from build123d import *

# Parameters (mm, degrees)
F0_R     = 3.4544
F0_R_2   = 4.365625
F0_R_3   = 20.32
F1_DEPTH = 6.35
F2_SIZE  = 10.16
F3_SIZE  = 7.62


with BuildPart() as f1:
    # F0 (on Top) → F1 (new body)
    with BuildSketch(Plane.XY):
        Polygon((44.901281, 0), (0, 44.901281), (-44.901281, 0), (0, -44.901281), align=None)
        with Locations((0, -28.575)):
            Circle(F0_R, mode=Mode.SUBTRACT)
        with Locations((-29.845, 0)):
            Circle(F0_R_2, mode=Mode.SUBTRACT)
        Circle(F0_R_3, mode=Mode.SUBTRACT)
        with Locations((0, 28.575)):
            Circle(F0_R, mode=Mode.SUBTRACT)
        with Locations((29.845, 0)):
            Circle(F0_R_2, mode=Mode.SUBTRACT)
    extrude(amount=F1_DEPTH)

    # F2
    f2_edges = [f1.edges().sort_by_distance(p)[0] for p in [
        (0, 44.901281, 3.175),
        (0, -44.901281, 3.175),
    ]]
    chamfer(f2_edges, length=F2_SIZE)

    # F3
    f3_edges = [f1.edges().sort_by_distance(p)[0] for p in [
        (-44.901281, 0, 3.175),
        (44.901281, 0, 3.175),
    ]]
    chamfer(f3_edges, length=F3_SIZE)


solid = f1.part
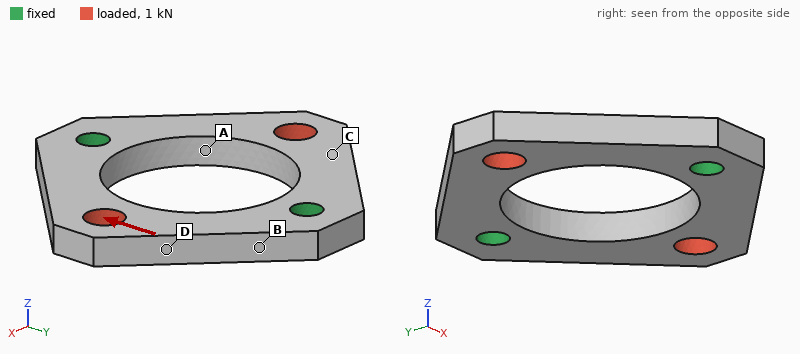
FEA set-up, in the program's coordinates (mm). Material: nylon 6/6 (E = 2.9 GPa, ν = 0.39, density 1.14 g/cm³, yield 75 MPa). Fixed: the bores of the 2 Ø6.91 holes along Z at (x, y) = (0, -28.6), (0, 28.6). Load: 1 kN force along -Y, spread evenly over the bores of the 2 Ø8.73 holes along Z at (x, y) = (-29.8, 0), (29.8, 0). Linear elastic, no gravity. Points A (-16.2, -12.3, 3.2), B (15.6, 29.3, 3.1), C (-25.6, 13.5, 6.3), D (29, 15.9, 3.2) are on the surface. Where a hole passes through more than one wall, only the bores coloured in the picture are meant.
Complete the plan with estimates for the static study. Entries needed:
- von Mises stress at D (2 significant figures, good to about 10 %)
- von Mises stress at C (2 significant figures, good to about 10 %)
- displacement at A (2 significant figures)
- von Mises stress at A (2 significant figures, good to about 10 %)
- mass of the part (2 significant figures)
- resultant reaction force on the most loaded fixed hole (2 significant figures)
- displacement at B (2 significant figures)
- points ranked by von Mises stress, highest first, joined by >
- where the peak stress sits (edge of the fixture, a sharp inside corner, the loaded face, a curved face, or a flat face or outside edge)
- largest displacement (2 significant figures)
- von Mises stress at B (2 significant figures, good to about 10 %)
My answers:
1.2 MPa
2.4 MPa
0.073 mm
8.9 MPa
17 g
500 N
0.050 mm
A > B > C > D
the loaded face
0.12 mm
5.5 MPa
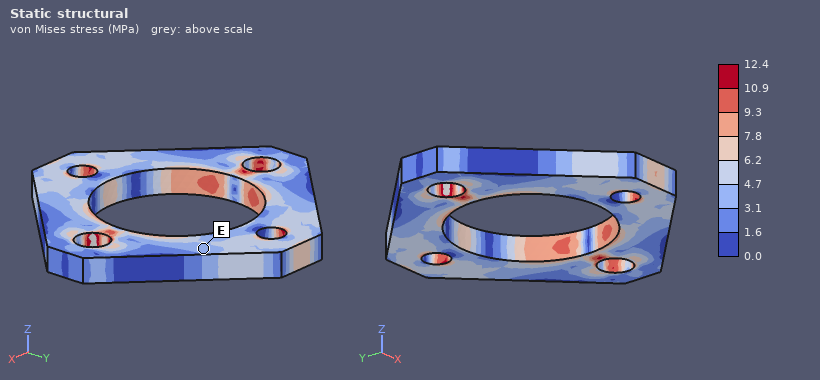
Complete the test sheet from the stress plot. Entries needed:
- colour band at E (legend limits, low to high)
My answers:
3.1 to 4.7 MPa
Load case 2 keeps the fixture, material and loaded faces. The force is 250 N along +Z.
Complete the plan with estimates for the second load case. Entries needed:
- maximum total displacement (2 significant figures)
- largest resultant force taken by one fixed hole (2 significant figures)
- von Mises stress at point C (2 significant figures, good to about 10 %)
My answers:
1.2 mm
130 N
6.2 MPa
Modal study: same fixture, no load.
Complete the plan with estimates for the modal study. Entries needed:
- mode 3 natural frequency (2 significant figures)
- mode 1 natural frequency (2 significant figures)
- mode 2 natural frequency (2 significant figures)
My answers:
3400 Hz
1100 Hz
1100 Hz
